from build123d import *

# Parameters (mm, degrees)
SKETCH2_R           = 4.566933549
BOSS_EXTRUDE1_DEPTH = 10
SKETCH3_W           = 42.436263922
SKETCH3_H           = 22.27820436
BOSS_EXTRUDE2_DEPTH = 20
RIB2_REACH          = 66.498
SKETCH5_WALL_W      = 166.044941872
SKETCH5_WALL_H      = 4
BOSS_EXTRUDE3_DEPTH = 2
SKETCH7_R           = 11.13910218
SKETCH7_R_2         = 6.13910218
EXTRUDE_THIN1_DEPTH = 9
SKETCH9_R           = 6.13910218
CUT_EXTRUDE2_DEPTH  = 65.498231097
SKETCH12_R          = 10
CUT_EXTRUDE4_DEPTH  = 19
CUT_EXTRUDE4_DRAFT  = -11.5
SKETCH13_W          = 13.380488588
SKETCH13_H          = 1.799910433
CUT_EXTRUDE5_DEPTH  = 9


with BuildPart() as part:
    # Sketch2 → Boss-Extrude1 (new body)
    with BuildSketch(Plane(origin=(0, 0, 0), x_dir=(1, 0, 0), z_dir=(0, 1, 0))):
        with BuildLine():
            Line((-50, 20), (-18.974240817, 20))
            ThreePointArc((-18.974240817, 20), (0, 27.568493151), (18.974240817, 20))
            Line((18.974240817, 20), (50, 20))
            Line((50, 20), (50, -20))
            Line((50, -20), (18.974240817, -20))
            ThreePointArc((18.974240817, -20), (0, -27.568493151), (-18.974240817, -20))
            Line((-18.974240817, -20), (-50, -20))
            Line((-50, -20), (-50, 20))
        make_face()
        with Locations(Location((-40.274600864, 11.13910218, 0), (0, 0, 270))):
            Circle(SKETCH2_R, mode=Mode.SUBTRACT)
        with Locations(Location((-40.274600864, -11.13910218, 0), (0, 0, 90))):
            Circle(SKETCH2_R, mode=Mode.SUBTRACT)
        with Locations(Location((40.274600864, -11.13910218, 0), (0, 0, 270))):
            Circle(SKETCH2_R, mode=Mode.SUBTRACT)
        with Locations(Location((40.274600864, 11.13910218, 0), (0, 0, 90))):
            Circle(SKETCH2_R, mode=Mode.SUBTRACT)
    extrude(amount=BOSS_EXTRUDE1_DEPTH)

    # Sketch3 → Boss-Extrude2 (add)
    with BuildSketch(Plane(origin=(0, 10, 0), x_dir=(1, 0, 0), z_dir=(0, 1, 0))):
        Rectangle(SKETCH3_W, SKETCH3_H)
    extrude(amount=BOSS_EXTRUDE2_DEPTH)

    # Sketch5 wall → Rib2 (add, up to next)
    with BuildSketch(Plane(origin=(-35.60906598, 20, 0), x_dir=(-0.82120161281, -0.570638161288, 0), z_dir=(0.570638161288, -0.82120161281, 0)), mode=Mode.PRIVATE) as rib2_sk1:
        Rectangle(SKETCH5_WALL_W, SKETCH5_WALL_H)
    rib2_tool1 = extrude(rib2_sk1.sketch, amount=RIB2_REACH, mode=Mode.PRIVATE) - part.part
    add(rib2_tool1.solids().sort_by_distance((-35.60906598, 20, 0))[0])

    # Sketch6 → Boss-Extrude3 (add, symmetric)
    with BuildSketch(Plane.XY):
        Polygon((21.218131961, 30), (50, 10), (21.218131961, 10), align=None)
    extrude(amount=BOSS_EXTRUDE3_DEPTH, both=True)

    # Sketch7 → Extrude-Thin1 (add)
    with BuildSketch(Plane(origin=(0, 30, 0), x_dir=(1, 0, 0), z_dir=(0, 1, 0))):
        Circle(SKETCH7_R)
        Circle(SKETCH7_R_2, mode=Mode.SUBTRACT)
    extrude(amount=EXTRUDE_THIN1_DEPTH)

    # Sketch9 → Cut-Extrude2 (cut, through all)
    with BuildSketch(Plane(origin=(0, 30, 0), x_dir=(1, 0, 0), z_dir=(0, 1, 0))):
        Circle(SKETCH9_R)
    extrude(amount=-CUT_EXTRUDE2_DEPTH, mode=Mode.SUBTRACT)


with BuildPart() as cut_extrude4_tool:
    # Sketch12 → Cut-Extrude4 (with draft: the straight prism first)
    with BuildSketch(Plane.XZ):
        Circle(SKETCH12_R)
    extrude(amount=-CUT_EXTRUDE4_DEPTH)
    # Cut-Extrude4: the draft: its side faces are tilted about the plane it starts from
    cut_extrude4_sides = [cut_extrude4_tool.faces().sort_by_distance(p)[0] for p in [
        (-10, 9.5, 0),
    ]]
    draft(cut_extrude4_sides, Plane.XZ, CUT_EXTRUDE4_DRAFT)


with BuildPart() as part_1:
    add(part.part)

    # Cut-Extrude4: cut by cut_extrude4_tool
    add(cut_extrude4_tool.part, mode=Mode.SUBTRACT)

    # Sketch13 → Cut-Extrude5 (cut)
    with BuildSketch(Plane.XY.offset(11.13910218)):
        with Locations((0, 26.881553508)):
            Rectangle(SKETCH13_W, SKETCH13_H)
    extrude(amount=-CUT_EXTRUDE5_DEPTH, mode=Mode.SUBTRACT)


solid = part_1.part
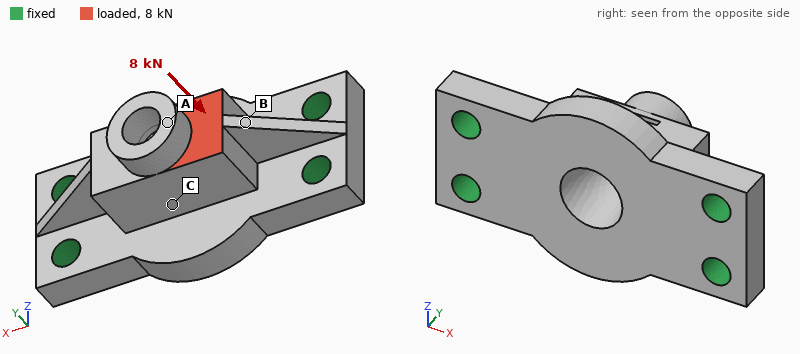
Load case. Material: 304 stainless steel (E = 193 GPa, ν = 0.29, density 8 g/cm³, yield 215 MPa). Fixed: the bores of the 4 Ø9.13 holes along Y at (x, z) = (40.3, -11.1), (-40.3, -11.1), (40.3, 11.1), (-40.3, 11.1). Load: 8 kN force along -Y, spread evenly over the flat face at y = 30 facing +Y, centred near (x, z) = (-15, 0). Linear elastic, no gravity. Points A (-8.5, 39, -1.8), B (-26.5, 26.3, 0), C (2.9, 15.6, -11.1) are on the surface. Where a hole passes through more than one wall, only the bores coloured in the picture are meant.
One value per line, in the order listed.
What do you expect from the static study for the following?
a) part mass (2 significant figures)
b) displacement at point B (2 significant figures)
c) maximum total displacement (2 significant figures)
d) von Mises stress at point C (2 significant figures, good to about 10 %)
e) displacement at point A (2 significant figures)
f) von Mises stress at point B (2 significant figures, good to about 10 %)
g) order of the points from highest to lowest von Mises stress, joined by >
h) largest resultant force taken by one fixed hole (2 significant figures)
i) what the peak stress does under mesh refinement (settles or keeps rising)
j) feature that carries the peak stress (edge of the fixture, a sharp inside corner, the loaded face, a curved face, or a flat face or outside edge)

480 g
7.4 µm
12 µm
21 MPa
11 µm
57 MPa
B > C > A
3.2 kN
keeps rising
edge of the fixture
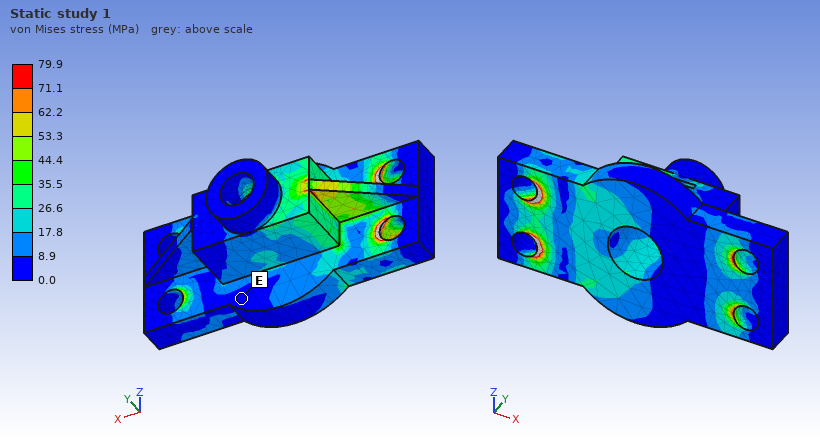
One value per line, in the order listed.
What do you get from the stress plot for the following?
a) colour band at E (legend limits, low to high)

0.0 to 8.9 MPa
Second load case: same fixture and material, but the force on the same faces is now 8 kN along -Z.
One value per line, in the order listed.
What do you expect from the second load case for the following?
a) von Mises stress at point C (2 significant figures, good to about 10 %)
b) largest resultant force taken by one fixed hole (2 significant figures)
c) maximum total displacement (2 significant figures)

51 MPa
5.3 kN
60 µm
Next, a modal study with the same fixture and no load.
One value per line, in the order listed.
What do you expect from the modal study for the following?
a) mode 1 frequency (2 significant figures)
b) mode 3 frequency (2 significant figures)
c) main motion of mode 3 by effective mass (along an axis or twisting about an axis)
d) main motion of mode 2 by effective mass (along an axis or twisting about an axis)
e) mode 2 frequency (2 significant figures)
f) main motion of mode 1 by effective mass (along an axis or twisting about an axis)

6100 Hz
14 kHz
along Z
along Y
8600 Hz
along Z
